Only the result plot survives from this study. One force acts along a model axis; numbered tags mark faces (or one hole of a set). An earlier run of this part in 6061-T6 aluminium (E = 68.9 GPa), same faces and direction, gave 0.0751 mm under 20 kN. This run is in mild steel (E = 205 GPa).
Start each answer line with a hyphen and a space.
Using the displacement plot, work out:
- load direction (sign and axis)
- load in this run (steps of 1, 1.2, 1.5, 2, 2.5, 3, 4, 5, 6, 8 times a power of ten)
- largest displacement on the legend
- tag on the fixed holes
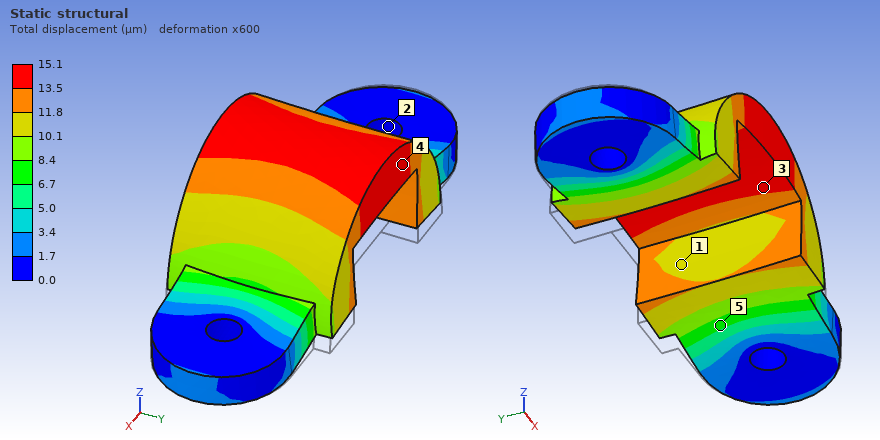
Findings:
- +Z
- 12 kN
- 15.1 µm
- 2
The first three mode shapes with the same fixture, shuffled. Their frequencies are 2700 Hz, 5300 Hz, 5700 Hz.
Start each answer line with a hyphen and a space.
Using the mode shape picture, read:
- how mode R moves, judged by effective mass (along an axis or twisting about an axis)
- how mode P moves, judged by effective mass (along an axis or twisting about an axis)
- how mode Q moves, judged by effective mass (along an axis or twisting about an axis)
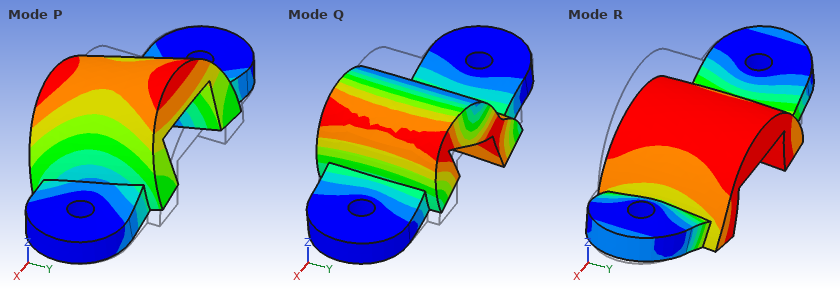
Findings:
- along Z
- along Y
- along X
